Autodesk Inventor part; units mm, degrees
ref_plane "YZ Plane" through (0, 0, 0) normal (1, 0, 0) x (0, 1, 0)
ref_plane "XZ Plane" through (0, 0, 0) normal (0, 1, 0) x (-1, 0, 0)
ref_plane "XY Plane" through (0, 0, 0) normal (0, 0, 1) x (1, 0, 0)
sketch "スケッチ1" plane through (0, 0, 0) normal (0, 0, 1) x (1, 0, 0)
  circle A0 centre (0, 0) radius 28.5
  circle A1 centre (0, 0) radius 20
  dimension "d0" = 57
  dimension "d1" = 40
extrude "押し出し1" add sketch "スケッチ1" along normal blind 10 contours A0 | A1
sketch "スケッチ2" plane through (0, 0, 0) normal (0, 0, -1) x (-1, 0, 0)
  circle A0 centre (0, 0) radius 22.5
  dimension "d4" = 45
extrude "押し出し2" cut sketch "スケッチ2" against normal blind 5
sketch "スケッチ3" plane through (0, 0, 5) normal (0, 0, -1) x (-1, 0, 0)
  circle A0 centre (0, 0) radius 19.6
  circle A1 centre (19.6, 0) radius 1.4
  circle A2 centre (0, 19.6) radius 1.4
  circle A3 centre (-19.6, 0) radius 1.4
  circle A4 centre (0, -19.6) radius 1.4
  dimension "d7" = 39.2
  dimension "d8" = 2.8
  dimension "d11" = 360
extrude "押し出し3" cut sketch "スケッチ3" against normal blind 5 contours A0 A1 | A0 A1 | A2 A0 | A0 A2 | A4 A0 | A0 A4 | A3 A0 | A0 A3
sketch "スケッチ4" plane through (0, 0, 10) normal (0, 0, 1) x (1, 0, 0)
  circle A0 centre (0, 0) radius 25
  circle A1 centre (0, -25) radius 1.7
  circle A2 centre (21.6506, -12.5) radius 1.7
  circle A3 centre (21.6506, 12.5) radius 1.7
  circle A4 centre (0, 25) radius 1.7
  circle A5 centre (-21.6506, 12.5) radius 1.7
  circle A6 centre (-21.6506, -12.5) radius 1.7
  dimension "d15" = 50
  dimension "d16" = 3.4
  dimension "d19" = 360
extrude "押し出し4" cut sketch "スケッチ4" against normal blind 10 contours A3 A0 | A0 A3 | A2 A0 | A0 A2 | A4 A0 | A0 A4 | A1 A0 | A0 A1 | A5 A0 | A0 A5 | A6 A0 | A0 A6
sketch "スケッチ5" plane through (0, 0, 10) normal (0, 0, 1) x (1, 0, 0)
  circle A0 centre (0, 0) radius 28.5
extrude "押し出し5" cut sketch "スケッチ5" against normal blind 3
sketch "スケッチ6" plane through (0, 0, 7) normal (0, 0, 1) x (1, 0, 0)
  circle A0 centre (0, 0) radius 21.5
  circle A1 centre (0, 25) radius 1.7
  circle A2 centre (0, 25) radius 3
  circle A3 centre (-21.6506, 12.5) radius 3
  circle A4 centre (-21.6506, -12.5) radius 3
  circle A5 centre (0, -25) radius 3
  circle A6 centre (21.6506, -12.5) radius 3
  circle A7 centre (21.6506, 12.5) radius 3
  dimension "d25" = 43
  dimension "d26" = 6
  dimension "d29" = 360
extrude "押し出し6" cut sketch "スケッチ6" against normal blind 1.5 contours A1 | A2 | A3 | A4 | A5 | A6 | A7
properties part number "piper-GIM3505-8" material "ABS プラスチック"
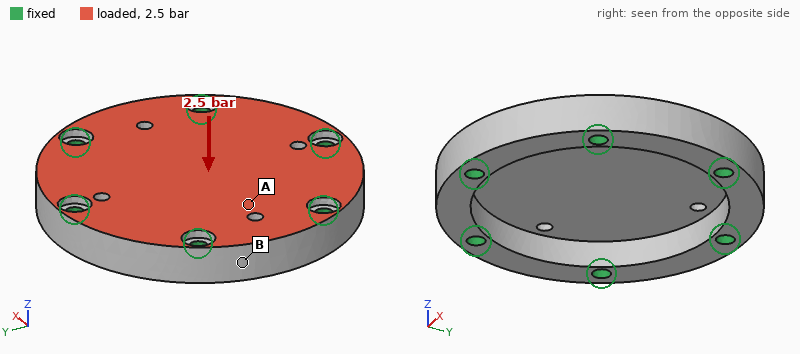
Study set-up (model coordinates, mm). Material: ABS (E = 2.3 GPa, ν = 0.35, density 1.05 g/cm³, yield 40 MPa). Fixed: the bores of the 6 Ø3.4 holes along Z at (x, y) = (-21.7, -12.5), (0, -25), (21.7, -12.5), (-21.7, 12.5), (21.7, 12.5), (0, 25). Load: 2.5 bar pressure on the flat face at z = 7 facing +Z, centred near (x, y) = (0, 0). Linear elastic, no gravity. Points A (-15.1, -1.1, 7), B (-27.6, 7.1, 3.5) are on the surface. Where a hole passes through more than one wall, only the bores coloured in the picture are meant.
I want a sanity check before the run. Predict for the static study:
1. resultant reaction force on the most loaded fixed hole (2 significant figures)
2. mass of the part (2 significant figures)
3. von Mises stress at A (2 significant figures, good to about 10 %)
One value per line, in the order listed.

120 N
9.8 g
9.1 MPa
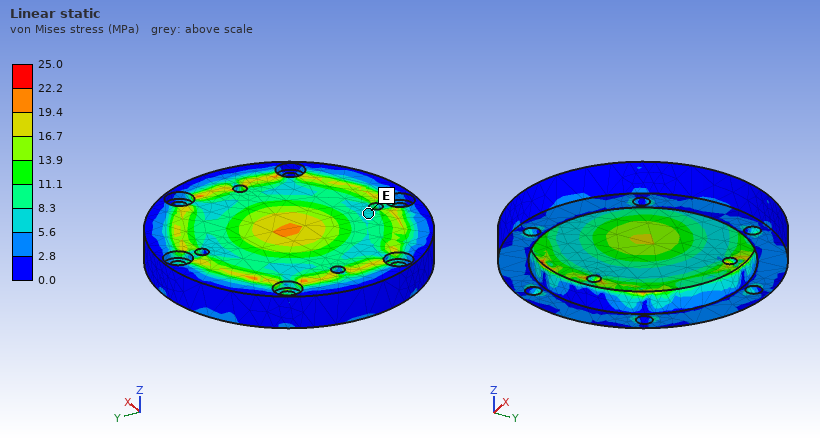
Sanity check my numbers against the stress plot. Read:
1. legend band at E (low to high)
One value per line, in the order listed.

5.6 to 8.3 MPa
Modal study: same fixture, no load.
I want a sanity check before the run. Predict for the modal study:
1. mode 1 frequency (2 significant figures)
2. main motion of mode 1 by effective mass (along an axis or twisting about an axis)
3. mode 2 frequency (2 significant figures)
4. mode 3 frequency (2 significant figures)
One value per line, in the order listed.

2500 Hz
along Z
4900 Hz
4900 Hz
